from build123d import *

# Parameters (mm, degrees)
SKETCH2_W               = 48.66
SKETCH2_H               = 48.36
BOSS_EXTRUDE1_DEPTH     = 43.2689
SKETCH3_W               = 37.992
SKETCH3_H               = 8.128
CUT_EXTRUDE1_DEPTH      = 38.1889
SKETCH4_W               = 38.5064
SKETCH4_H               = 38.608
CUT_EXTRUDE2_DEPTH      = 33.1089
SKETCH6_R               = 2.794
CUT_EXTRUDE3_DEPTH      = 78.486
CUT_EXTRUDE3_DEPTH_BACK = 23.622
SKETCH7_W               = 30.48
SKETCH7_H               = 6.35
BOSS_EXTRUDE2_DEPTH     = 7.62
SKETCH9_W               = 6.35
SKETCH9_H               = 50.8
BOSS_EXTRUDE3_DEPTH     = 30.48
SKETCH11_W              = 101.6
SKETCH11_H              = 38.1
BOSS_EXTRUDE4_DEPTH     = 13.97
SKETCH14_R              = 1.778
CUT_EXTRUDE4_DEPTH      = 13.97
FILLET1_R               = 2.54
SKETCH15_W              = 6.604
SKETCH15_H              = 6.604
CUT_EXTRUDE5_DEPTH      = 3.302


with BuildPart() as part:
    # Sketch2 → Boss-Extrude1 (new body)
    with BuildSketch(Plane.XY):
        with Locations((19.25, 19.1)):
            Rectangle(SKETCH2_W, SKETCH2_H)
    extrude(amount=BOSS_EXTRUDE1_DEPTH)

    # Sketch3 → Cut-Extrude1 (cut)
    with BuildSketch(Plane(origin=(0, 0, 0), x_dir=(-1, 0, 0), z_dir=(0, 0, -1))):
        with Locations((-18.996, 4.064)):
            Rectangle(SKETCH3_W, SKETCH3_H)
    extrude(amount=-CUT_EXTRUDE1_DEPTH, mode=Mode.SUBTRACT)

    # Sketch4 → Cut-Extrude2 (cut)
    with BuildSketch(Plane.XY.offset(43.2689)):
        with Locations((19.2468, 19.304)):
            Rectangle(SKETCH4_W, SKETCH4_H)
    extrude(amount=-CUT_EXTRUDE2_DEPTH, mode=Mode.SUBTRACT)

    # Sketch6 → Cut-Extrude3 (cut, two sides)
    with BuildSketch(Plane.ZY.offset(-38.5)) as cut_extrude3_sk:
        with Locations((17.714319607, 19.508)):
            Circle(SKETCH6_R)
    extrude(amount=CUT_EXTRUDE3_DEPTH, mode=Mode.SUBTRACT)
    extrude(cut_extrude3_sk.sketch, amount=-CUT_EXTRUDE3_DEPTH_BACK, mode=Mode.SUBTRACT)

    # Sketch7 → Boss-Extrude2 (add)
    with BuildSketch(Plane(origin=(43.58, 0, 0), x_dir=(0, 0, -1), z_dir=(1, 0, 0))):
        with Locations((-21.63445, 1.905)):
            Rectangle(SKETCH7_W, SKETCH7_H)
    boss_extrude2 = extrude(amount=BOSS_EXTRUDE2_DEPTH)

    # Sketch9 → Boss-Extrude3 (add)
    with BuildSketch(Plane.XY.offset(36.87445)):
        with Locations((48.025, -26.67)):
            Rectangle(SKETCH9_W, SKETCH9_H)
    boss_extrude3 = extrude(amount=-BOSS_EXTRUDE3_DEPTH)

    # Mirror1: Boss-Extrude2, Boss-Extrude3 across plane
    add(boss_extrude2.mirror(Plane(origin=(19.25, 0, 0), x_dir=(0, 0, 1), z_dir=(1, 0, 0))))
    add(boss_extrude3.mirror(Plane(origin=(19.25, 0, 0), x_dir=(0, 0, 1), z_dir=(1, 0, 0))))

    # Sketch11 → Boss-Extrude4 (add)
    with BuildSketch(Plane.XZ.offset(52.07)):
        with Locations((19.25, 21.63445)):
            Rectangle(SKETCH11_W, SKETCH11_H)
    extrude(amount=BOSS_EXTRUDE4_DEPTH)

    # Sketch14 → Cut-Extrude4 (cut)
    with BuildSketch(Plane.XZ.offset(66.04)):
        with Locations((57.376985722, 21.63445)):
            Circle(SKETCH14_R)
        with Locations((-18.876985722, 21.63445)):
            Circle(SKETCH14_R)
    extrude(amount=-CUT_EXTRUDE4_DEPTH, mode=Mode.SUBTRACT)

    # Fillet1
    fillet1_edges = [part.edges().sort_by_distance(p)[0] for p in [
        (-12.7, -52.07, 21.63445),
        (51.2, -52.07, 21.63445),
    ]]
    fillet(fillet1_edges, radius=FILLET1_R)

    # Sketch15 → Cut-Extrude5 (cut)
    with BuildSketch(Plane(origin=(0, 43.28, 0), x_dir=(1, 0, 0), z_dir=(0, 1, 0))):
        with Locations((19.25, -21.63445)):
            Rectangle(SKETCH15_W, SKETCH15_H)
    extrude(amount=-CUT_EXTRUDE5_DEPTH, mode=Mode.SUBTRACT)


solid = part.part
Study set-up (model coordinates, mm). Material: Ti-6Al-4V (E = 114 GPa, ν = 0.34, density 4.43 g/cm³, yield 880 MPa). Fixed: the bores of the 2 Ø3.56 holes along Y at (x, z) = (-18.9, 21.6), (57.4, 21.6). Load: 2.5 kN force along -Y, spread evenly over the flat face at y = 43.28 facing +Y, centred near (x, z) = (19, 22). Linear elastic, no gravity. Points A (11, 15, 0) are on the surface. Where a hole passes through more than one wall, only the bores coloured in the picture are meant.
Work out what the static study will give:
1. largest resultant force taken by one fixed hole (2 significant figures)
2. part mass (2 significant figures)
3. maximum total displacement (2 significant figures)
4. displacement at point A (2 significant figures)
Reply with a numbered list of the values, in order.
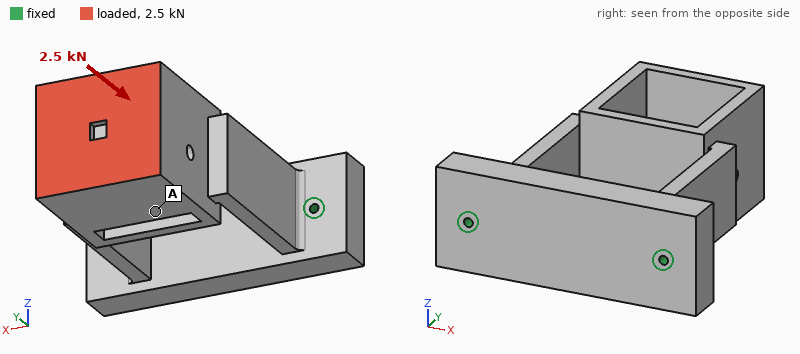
1. 1.3 kN
2. 560 g
3. 28 µm
4. 7.8 µm
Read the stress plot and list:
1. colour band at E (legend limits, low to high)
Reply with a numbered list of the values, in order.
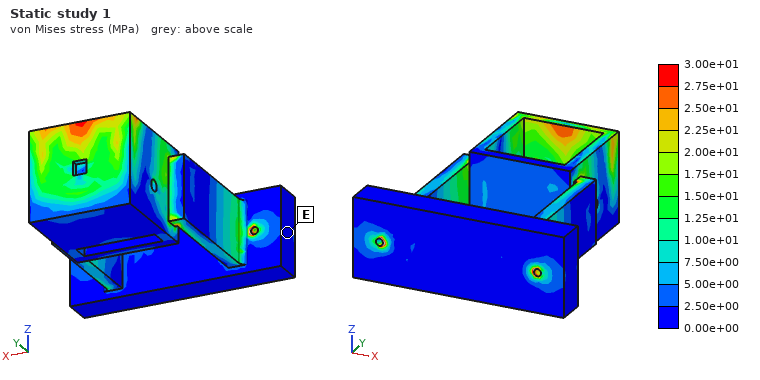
1. 0.00e+00 to 2.50e+00 MPa
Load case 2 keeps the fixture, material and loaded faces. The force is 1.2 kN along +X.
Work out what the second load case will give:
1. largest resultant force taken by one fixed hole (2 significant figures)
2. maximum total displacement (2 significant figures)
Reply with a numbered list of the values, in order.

1. 1.7 kN
2. 0.21 mm
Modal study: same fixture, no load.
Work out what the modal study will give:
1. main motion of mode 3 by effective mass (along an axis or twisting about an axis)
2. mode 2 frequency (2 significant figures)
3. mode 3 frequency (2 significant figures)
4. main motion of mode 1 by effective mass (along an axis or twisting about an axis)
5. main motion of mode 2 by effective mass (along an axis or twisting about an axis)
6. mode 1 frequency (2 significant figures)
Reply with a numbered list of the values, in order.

1. twisting about Y
2. 1000 Hz
3. 2400 Hz
4. along X
5. along Z
6. 890 Hz
